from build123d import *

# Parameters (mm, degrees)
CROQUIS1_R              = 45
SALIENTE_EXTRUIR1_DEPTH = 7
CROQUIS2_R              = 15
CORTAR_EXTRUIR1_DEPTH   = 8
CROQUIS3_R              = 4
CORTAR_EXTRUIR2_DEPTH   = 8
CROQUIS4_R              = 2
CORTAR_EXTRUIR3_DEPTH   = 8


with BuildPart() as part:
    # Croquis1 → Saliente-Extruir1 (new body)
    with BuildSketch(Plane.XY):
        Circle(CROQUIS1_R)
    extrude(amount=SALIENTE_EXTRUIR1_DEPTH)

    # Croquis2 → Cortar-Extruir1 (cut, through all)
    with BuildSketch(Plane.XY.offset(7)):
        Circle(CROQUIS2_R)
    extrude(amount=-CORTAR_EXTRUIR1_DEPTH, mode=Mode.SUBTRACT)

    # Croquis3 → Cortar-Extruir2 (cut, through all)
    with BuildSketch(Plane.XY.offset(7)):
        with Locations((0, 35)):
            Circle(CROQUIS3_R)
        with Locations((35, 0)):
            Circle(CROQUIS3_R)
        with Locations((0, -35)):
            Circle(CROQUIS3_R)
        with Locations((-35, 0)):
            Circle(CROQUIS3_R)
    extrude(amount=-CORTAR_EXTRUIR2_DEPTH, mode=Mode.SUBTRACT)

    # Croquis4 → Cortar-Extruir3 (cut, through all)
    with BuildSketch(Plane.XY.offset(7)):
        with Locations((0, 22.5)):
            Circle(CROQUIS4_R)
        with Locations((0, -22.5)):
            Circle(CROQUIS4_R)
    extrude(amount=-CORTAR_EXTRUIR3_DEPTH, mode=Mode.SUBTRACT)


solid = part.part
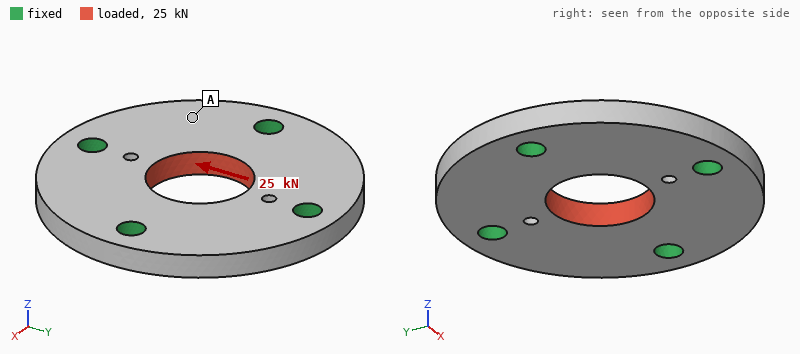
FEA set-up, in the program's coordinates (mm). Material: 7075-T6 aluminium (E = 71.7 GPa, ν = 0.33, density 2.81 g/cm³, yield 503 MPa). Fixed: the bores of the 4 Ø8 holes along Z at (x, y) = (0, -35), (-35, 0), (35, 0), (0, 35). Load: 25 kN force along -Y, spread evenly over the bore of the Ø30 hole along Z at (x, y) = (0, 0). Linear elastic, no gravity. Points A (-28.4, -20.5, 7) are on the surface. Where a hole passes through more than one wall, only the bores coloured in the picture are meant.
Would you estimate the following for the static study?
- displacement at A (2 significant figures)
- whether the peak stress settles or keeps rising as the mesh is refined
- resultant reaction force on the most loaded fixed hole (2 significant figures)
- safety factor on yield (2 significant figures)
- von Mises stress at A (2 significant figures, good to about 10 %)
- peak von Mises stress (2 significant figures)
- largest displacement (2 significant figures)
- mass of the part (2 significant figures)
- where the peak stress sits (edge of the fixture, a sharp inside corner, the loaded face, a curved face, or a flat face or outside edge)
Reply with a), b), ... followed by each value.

a) 9.0 µm
b) settles
c) 7.4 kN
d) 3.1
e) 15 MPa
f) 160 MPa
g) 19 µm
h) 110 g
i) a curved face
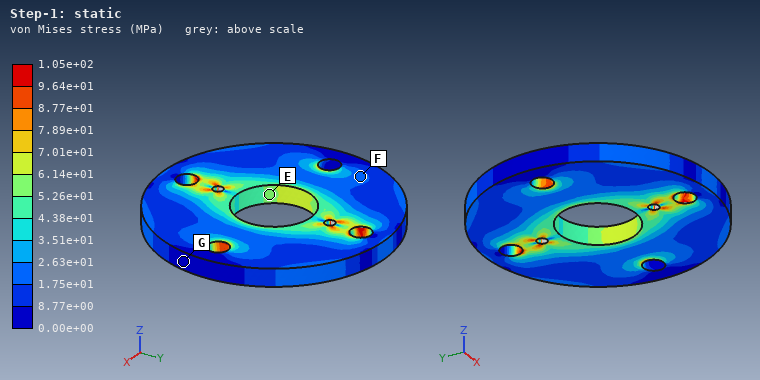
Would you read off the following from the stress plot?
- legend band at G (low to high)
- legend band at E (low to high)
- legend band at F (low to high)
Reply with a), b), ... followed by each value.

a) 0.00e+00 to 8.77e+00 MPa
b) 5.26e+01 to 6.14e+01 MPa
c) 1.75e+01 to 2.63e+01 MPa
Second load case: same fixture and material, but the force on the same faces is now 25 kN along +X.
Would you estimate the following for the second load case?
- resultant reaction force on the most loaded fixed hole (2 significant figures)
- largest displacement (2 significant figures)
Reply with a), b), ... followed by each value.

a) 7.6 kN
b) 19 µm
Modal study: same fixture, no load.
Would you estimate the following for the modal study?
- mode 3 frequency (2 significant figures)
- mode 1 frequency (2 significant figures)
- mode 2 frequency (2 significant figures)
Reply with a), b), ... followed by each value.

a) 11 kHz
b) 11 kHz
c) 11 kHz
